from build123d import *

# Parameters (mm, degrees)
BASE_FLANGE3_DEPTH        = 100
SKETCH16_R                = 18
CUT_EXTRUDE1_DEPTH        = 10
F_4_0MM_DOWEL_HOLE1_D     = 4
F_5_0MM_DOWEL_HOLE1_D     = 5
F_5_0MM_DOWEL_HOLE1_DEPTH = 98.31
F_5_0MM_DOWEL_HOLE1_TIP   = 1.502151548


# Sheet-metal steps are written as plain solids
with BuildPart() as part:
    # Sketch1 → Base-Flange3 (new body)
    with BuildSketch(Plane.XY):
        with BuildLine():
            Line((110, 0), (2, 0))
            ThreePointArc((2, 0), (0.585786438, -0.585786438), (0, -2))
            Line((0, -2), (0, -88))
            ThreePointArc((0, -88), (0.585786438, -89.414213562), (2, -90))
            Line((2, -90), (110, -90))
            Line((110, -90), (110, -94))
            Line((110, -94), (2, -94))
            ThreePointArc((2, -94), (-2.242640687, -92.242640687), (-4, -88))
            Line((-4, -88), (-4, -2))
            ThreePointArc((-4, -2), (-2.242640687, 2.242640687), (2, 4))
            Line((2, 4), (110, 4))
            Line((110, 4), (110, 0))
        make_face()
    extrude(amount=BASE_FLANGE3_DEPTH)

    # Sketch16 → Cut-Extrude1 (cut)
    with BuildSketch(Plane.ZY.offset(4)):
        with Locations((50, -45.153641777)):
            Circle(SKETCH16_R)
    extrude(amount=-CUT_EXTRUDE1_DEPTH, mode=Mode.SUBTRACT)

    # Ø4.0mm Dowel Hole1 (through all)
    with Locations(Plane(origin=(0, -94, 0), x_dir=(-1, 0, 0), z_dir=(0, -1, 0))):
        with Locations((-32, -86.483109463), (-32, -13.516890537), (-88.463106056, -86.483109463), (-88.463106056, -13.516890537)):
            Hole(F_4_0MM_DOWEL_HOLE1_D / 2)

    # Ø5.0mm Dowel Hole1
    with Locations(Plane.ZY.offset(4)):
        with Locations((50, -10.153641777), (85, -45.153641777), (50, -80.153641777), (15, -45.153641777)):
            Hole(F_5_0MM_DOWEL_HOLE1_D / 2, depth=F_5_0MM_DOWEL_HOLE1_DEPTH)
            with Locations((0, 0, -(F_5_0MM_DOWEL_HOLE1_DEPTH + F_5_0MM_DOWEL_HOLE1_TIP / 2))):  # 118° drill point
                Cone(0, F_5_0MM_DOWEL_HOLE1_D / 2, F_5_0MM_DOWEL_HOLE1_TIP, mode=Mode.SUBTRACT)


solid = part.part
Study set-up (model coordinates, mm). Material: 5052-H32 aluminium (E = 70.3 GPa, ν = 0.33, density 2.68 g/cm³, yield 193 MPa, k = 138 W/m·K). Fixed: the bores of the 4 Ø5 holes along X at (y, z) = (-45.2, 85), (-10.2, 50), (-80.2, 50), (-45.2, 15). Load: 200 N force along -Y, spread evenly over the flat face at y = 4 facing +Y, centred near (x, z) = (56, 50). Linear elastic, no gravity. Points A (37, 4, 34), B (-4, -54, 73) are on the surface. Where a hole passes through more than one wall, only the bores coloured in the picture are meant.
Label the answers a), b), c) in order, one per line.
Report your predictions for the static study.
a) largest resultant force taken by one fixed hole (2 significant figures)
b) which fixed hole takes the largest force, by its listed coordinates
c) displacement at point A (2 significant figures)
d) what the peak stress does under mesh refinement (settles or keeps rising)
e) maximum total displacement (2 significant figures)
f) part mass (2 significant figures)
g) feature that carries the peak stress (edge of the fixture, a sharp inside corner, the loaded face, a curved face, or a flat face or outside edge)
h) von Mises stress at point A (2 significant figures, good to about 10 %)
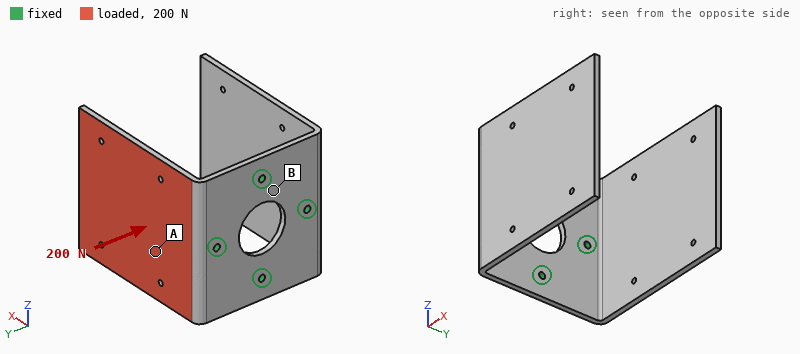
a) 240 N
b) (-10.2, 50)
c) 0.34 mm
d) keeps rising
e) 1.4 mm
f) 320 g
g) edge of the fixture
h) 17 MPa
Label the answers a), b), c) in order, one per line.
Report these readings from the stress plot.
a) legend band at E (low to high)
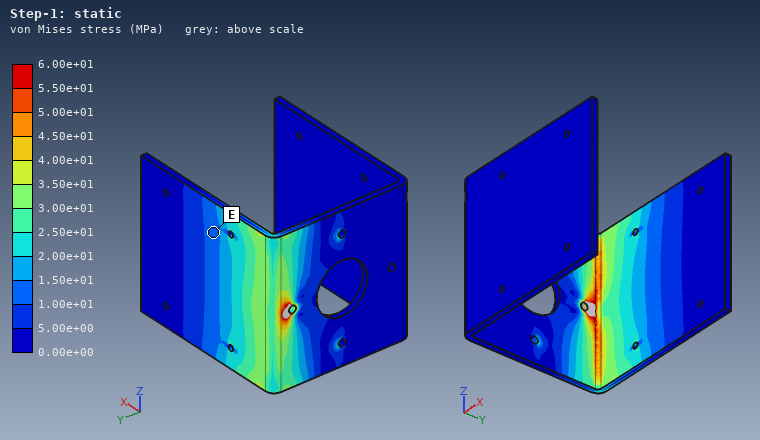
a) 1.00e+01 to 1.50e+01 MPa
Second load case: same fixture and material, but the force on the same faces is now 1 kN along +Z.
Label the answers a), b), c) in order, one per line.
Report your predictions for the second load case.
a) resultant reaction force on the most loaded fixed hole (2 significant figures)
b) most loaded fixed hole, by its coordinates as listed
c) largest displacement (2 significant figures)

a) 820 N
b) (-10.2, 50)
c) 1.6 mm
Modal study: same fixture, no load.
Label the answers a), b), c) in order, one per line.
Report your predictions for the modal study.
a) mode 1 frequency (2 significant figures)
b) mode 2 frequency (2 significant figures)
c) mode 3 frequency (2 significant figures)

a) 220 Hz
b) 220 Hz
c) 410 Hz
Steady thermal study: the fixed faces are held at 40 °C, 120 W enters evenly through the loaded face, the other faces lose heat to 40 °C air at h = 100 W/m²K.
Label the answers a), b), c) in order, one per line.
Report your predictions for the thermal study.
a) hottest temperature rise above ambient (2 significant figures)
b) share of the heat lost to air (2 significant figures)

a) 68 K
b) 66 %
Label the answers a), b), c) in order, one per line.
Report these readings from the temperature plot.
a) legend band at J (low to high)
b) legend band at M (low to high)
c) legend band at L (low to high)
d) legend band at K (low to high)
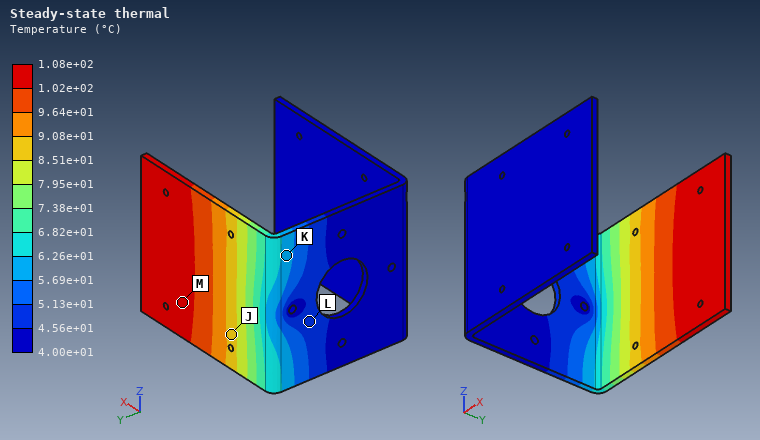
a) 8.51e+01 to 9.08e+01 °C
b) 1.02e+02 to 1.08e+02 °C
c) 4.56e+01 to 5.13e+01 °C
d) 5.69e+01 to 6.26e+01 °C
